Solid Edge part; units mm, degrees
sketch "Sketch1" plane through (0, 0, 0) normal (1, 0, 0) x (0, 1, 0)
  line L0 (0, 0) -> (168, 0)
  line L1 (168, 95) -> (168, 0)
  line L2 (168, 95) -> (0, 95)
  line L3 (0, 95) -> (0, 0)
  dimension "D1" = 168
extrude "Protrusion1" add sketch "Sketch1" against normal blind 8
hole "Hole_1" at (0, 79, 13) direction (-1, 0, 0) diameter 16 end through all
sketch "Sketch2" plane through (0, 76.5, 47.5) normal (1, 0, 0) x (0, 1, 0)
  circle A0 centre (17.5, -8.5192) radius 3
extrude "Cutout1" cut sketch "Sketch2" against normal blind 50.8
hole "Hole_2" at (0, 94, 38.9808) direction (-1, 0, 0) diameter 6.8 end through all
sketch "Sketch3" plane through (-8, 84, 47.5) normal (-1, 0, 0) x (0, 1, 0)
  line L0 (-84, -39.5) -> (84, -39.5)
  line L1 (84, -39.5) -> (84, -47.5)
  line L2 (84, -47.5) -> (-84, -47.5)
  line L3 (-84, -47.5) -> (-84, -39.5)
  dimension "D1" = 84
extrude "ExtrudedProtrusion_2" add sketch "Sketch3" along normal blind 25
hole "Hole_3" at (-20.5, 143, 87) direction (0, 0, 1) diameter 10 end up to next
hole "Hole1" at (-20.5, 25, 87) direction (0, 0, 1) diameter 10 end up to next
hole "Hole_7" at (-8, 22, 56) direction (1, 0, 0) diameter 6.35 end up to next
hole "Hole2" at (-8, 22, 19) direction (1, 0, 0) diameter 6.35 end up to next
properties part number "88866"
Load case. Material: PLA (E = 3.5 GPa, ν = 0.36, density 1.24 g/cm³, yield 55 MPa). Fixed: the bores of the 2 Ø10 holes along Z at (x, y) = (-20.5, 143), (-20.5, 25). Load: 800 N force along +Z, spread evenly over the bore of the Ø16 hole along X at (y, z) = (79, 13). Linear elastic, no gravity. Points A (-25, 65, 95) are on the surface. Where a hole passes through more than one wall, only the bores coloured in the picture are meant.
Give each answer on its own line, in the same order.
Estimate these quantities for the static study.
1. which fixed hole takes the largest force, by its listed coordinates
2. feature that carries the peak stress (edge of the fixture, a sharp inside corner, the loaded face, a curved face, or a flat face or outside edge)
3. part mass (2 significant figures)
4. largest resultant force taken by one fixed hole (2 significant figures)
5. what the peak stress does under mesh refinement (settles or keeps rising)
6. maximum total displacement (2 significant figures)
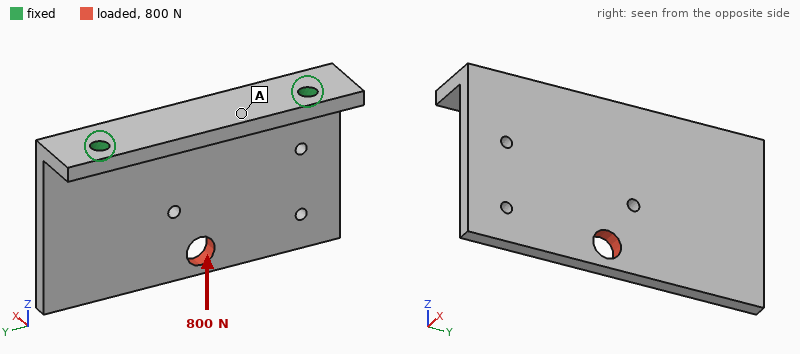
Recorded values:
(-20.5, 25)
edge of the fixture
200 g
440 N
keeps rising
0.64 mm
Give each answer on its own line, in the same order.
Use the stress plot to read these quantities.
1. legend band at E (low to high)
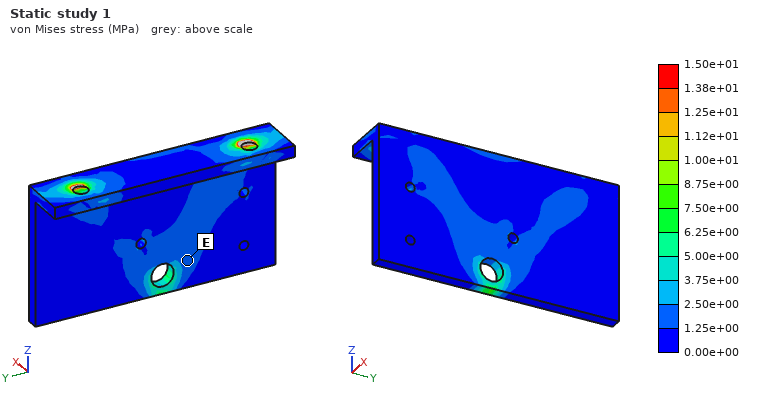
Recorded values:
1.25e+00 to 2.50e+00 MPa
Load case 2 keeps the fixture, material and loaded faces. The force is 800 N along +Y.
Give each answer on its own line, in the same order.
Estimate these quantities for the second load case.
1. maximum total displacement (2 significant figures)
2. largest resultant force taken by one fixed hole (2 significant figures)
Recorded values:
0.44 mm
660 N
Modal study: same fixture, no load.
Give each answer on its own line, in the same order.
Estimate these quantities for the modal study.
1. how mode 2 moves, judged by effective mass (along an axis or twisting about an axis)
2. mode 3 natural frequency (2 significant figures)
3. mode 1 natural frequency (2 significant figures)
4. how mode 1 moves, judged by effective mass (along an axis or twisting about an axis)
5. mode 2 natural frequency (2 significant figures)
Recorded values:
twisting about Z
770 Hz
190 Hz
along X
360 Hz
